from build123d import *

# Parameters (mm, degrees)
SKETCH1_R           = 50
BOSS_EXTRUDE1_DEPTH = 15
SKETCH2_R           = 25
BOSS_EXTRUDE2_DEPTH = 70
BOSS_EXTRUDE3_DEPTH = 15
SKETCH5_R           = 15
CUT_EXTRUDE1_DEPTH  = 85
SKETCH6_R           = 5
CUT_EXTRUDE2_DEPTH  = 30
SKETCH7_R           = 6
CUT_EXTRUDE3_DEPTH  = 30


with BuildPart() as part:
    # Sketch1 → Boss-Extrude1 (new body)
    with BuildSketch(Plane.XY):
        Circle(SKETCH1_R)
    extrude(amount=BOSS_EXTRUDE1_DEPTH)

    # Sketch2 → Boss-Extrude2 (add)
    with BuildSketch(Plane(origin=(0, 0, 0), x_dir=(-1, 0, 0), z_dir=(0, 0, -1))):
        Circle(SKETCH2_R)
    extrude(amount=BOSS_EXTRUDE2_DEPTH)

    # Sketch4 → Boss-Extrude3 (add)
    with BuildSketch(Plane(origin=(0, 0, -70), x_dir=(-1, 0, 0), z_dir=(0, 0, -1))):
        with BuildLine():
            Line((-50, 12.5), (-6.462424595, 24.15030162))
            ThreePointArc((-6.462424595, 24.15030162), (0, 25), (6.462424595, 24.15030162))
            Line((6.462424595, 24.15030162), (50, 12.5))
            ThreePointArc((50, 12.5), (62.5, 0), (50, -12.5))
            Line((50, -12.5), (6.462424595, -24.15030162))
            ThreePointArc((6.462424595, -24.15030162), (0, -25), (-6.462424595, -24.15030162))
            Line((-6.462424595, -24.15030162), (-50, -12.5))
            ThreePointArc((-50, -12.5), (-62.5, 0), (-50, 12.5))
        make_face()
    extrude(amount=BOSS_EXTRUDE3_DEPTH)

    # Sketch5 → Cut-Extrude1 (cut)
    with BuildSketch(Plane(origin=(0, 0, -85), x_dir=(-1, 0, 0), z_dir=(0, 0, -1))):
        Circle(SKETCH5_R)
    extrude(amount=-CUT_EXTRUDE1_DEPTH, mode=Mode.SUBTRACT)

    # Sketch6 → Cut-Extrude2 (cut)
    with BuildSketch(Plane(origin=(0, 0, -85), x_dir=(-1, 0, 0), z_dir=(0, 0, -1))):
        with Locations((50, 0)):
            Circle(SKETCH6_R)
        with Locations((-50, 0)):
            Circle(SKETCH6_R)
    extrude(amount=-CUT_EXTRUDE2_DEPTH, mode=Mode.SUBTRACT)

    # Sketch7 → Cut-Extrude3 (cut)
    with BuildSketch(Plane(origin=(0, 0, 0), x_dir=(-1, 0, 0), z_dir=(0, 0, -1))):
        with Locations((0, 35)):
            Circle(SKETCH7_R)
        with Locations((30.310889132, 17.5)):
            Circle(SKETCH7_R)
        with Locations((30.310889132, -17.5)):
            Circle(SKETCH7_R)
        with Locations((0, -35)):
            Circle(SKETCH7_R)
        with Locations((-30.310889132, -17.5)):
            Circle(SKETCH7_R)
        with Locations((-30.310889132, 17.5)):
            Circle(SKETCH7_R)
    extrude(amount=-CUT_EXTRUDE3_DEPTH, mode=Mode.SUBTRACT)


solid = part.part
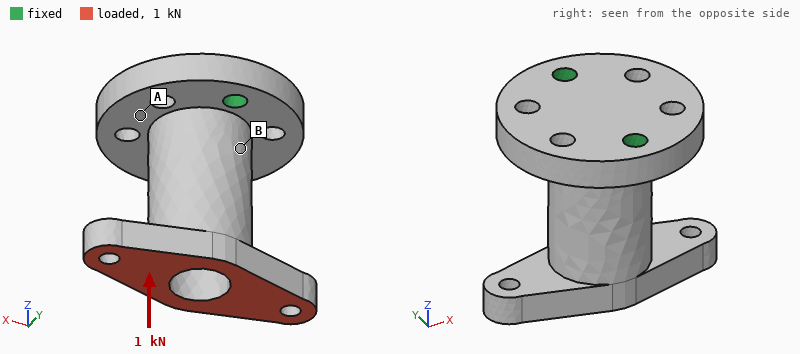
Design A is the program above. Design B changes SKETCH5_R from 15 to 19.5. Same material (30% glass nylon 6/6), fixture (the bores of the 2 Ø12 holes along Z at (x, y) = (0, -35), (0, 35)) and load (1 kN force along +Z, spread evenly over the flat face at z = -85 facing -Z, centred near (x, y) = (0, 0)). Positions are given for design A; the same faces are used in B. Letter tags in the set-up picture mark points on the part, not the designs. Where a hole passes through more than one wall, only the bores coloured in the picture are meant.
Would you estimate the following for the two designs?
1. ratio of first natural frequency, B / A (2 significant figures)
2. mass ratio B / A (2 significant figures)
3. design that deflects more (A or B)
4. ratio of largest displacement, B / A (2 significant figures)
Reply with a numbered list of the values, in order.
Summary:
1. 1.1
2. 0.83
3. B
4. 1.7
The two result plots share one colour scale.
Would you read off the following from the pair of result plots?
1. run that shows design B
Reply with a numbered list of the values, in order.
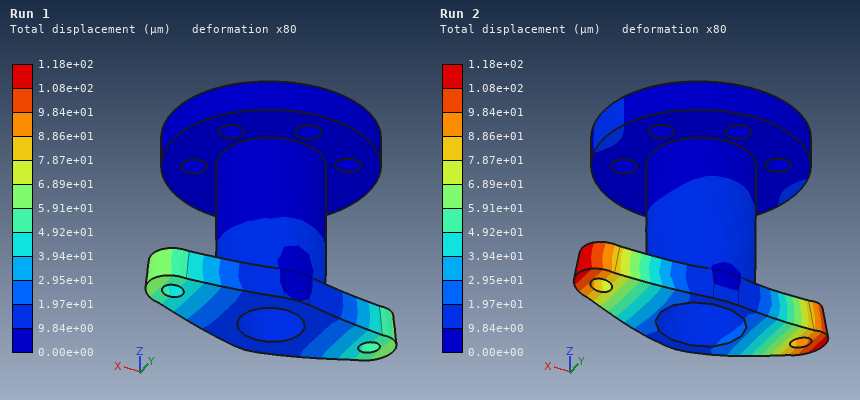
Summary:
1. Run 2
